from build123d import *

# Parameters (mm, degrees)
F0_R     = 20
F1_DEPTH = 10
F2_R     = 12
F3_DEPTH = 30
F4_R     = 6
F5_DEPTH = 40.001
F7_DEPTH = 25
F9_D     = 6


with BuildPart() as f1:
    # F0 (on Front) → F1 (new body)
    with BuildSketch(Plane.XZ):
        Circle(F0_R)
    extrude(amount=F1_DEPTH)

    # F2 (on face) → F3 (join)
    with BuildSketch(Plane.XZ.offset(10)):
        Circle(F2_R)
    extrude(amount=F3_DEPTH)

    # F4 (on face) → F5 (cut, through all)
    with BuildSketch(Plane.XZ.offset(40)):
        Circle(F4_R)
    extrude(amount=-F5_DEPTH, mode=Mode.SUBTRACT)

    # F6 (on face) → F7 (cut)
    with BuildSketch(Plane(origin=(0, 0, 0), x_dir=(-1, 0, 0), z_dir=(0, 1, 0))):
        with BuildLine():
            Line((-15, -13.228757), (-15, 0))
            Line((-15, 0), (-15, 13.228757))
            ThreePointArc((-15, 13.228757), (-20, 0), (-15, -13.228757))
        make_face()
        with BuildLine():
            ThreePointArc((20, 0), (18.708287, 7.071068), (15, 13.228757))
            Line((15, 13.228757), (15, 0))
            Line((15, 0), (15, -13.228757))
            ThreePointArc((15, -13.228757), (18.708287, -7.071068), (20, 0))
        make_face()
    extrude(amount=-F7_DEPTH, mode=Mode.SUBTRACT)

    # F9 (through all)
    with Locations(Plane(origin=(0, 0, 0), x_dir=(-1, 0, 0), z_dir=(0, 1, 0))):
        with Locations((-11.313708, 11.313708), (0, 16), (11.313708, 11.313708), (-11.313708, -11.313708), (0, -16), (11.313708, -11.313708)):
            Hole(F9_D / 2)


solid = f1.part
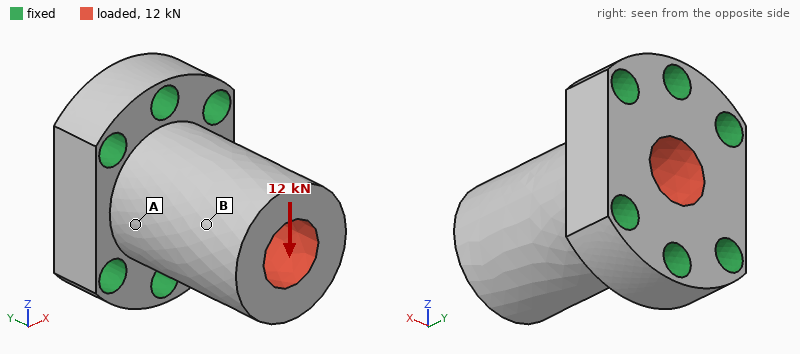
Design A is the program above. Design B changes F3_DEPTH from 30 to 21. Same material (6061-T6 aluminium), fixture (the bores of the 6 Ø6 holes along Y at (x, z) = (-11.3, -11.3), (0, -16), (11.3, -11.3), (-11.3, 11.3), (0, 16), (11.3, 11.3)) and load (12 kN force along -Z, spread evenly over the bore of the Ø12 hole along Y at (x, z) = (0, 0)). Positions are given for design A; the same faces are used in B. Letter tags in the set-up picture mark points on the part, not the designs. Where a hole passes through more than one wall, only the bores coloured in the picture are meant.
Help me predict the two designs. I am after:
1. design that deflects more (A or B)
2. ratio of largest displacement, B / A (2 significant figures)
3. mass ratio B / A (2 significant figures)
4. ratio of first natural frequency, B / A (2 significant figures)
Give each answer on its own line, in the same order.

A
0.48
0.83
1.6
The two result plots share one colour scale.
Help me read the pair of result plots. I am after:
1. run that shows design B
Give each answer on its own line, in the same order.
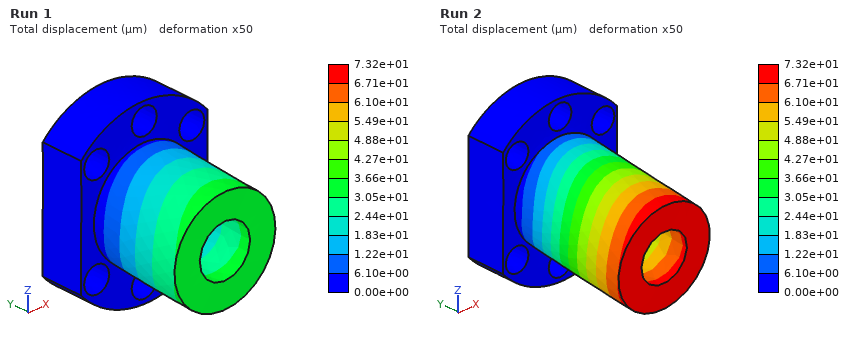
Run 1
